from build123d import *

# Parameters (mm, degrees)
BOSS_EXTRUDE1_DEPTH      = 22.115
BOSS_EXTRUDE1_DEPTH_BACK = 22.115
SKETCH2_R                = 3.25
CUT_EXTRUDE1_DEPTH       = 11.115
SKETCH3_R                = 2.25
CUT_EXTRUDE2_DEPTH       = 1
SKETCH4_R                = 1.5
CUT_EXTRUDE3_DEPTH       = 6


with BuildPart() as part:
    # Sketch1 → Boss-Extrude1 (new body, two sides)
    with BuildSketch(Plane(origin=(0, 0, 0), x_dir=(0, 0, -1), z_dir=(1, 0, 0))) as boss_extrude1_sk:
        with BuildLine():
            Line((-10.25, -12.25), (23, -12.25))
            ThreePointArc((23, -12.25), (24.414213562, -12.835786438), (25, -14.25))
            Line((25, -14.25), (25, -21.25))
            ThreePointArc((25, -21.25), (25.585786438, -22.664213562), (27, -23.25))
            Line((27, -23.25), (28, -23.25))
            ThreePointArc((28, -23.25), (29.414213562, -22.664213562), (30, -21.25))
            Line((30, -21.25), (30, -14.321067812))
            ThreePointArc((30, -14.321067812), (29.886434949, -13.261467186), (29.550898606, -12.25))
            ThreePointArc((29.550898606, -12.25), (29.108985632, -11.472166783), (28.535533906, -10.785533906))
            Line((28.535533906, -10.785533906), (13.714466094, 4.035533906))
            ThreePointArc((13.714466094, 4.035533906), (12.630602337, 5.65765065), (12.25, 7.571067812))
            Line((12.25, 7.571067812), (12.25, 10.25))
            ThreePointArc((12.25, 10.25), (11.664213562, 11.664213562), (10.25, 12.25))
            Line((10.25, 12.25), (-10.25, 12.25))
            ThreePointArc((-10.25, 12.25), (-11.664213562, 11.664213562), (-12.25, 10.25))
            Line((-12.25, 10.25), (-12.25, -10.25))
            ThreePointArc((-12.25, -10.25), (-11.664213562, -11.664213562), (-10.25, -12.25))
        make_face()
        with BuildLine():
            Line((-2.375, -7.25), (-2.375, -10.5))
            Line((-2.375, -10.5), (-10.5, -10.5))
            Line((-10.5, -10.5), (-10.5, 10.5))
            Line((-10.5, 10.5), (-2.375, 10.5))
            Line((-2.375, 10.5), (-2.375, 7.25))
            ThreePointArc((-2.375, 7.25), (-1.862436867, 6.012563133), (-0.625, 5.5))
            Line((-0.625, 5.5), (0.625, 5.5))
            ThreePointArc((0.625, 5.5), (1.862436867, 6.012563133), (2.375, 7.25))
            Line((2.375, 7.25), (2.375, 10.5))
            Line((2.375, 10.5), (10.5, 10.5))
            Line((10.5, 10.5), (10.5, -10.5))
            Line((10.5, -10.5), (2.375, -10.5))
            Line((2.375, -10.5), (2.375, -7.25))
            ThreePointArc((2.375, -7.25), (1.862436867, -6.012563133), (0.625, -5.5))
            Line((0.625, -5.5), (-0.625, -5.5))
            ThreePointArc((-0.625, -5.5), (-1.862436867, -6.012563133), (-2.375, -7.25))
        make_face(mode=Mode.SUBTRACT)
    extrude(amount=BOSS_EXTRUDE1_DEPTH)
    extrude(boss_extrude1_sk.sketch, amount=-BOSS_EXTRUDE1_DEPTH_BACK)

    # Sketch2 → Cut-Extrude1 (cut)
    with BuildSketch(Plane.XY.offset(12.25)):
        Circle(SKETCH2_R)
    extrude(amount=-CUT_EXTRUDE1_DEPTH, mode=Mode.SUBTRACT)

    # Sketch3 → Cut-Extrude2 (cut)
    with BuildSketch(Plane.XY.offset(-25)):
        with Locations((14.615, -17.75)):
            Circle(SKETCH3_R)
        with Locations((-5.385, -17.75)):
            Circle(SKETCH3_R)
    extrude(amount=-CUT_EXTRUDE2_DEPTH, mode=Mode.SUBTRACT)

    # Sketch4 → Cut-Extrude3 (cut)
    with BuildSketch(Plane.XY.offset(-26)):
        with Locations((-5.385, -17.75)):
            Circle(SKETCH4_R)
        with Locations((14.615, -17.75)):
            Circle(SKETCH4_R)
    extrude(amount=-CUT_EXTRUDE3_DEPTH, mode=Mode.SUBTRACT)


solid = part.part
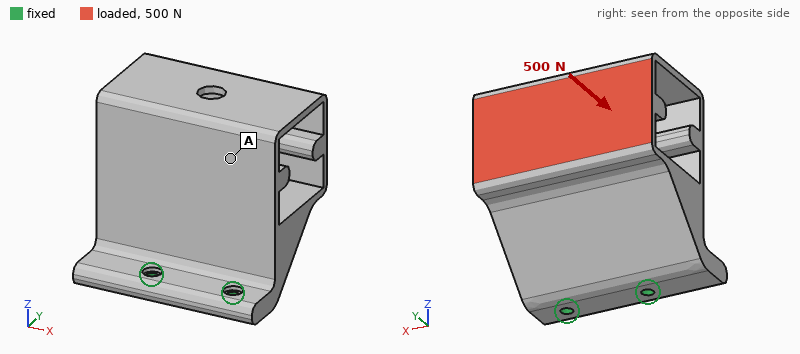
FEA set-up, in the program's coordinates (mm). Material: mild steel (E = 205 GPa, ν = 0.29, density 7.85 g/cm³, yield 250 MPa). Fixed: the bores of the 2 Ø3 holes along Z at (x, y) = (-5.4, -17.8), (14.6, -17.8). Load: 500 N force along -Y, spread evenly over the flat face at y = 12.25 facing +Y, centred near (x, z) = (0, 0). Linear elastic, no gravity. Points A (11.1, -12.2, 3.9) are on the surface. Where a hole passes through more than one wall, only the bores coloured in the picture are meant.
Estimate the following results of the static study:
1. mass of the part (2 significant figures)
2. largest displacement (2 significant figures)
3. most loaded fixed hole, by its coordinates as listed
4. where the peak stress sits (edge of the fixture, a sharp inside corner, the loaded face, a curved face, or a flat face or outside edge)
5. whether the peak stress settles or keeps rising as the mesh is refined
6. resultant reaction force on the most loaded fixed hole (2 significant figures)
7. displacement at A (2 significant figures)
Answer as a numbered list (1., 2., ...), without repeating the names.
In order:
1. 140 g
2. 0.17 mm
3. (-5.4, -17.8)
4. edge of the fixture
5. keeps rising
6. 350 N
7. 0.11 mm
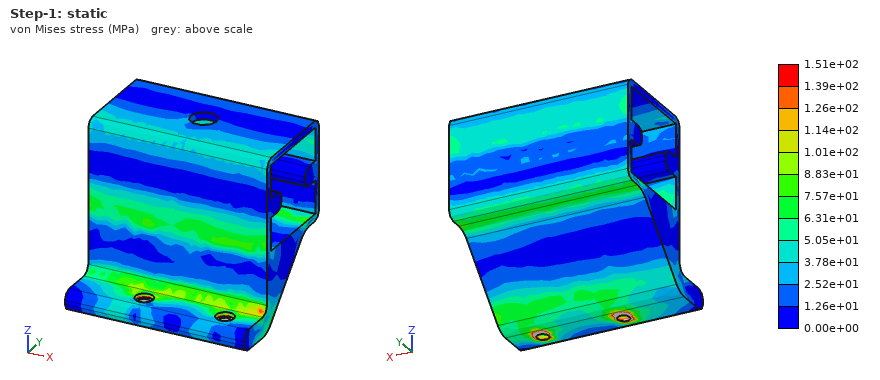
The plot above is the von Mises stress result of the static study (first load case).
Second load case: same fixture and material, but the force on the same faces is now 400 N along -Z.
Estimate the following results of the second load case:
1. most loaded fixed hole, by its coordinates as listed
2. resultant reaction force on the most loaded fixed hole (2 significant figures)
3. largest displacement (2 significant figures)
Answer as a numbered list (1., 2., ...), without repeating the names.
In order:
1. (-5.4, -17.8)
2. 290 N
3. 0.11 mm
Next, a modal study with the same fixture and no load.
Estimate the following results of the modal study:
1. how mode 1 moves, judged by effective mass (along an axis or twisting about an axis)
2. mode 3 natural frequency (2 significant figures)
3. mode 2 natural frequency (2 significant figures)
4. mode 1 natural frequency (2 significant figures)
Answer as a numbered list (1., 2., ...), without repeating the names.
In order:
1. along Y
2. 3800 Hz
3. 3500 Hz
4. 1100 Hz
